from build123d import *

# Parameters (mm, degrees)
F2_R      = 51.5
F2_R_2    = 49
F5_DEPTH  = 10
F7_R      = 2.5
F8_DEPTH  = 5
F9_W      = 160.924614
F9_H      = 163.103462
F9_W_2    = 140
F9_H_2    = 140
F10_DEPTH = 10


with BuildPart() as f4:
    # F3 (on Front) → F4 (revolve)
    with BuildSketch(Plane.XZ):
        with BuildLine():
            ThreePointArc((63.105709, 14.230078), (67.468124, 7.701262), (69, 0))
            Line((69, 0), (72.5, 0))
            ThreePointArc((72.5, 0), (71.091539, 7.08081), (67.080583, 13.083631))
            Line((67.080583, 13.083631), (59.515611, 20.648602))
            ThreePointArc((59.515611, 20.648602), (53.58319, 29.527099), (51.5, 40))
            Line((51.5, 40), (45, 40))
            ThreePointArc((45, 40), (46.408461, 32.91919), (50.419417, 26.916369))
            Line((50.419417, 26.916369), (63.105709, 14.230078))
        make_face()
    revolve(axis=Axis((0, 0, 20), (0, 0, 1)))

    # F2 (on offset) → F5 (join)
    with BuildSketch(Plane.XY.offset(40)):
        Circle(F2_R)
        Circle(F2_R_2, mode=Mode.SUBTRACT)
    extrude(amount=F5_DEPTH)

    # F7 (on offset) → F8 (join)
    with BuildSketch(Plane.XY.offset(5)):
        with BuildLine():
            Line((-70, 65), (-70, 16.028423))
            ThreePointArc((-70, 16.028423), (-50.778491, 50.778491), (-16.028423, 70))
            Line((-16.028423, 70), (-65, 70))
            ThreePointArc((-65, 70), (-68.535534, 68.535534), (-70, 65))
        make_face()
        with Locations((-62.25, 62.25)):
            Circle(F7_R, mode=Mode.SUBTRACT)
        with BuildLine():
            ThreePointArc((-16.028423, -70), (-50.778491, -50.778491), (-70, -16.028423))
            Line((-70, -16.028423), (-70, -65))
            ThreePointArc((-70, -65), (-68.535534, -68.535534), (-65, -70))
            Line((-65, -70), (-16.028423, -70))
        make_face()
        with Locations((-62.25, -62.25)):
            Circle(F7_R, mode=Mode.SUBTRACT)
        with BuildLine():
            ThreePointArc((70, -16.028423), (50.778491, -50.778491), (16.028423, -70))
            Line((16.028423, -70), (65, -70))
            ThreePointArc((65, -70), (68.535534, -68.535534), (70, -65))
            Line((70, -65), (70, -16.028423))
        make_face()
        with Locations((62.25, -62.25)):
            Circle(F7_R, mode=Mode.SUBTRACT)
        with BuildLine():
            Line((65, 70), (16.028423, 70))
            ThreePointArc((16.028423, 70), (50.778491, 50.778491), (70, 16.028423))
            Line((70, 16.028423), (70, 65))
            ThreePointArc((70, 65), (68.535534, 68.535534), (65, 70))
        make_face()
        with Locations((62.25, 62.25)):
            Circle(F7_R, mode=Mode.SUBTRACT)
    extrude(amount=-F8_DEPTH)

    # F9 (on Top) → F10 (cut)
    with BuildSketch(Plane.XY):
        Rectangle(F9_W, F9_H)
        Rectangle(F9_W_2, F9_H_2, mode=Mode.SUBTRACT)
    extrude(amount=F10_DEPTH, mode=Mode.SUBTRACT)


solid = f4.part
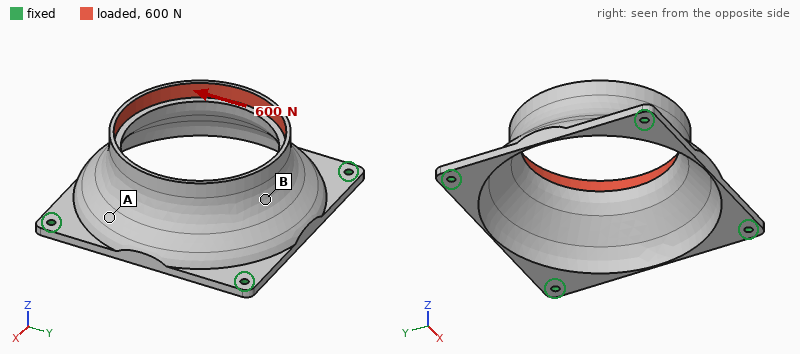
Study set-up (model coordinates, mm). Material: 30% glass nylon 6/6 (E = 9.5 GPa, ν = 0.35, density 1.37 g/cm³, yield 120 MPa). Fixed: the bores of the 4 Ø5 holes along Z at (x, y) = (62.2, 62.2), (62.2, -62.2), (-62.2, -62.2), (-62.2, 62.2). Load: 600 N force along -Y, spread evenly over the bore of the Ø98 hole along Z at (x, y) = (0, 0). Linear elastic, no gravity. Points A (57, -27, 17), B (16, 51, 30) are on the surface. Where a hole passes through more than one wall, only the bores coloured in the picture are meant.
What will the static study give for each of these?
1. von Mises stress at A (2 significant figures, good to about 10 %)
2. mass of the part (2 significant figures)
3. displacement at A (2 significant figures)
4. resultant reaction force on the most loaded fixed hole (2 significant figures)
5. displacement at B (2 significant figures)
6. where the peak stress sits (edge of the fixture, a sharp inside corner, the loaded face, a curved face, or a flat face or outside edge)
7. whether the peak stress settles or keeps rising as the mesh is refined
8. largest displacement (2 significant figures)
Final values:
2.5 MPa
110 g
34 µm
200 N
58 µm
edge of the fixture
keeps rising
91 µm
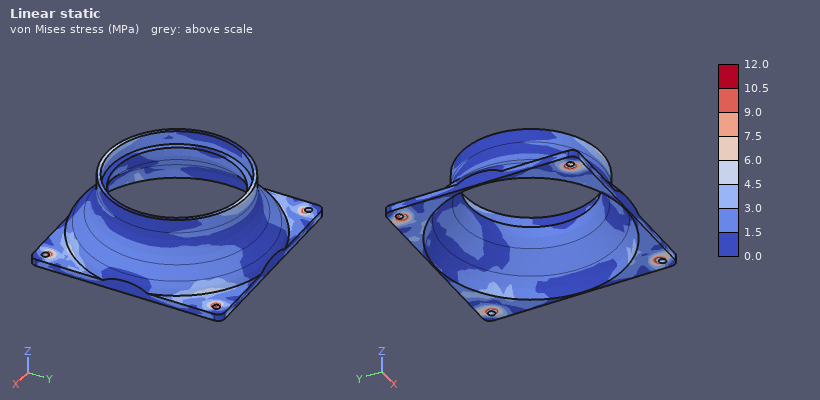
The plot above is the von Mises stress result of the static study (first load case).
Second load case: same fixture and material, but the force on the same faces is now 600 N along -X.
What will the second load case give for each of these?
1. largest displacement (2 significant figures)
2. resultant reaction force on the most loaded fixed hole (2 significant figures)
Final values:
91 µm
200 N
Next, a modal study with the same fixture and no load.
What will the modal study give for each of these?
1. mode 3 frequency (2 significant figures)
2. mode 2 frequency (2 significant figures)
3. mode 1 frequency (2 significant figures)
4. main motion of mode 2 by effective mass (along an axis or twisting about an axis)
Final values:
1700 Hz
1600 Hz
1200 Hz
along Z
